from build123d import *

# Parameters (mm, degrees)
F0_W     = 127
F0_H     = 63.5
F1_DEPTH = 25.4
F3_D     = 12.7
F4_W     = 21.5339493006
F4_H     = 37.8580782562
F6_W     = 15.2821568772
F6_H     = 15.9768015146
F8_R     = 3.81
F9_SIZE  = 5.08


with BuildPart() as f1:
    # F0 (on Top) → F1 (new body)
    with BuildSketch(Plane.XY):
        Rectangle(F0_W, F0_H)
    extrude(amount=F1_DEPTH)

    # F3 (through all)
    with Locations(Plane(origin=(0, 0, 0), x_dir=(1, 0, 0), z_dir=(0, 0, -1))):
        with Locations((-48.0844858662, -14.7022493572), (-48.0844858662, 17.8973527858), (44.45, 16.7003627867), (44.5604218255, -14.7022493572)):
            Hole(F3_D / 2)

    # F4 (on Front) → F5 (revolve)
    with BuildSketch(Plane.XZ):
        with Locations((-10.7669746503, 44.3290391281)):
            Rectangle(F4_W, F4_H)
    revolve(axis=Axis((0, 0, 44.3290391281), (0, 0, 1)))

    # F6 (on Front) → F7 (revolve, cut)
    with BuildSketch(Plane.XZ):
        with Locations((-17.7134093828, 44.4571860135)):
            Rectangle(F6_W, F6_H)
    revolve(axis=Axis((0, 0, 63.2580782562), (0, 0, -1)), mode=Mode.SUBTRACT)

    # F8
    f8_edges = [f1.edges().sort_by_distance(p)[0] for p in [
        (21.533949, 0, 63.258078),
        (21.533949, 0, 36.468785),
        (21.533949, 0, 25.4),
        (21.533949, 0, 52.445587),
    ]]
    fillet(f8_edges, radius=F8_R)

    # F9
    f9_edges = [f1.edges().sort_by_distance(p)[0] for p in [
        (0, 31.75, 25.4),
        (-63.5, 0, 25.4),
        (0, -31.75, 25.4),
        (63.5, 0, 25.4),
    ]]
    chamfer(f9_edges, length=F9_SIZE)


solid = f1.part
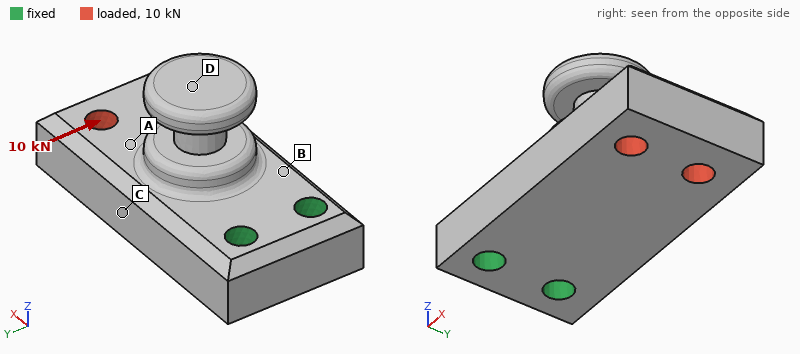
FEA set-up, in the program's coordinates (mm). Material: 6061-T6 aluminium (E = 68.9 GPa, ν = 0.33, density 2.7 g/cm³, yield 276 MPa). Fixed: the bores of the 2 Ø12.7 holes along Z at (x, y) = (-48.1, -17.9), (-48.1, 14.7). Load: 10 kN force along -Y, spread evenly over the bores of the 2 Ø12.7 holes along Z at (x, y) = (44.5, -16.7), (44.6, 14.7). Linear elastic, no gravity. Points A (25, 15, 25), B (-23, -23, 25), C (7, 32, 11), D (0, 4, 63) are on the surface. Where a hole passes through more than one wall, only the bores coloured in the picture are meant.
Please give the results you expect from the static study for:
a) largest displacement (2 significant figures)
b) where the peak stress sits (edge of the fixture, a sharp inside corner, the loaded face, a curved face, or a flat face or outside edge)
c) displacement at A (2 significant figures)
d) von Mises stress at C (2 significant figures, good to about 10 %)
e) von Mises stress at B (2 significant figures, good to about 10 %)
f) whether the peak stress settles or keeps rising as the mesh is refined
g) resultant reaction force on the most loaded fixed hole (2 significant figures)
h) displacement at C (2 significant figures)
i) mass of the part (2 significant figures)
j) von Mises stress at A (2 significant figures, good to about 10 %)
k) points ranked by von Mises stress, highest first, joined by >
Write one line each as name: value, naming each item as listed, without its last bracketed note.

largest displacement: 0.13 mm
where the peak stress sits: edge of the fixture
displacement at A: 0.071 mm
von Mises stress at C: 23 MPa
von Mises stress at B: 34 MPa
whether the peak stress settles or keeps rising as the mesh is refined: keeps rising
resultant reaction force on the most loaded fixed hole: 23 kN
displacement at C: 0.058 mm
mass of the part: 600 g
von Mises stress at A: 15 MPa
points ranked by von Mises stress, highest first, joined by >: B > C > A > D
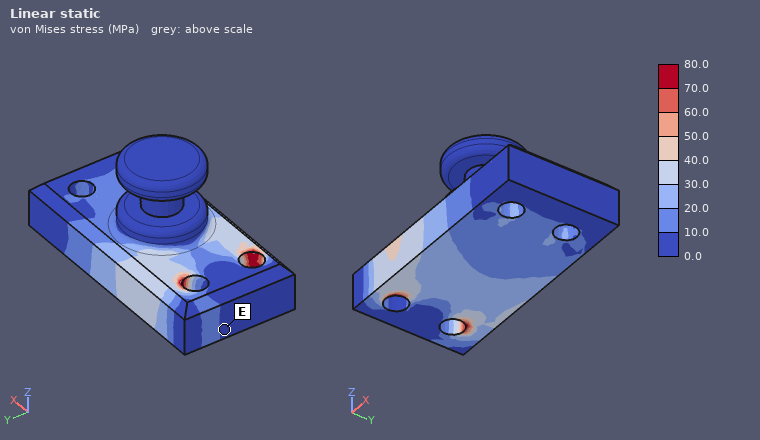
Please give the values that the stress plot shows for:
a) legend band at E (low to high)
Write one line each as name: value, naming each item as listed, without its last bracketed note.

legend band at E: 0.0 to 10.0 MPa
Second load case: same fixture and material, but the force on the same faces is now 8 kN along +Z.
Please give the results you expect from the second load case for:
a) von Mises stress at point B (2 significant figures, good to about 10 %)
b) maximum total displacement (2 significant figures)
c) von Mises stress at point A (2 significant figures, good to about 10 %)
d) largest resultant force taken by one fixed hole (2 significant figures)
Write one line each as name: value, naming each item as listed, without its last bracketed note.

von Mises stress at point B: 76 MPa
maximum total displacement: 0.41 mm
von Mises stress at point A: 24 MPa
largest resultant force taken by one fixed hole: 4.1 kN
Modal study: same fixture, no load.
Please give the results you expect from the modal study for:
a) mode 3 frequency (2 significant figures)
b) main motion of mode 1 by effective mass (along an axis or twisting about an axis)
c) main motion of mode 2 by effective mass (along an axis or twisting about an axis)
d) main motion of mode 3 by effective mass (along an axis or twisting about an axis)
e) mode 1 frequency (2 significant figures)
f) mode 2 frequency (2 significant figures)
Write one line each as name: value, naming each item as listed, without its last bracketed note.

mode 3 frequency: 4200 Hz
main motion of mode 1 by effective mass: along Z
main motion of mode 2 by effective mass: along Y
main motion of mode 3 by effective mass: twisting about X
mode 1 frequency: 1700 Hz
mode 2 frequency: 3400 Hz
